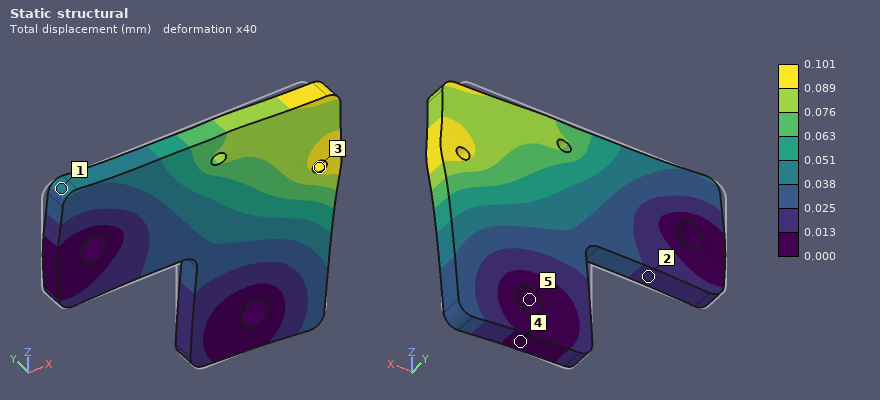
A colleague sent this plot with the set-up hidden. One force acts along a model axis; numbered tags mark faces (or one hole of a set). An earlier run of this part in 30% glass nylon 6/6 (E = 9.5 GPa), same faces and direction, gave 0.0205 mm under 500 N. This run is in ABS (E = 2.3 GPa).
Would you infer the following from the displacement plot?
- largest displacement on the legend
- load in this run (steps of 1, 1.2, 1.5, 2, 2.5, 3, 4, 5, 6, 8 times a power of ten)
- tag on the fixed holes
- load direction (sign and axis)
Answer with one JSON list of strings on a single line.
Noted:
["0.101 mm", "600 N", "5", "+X"]
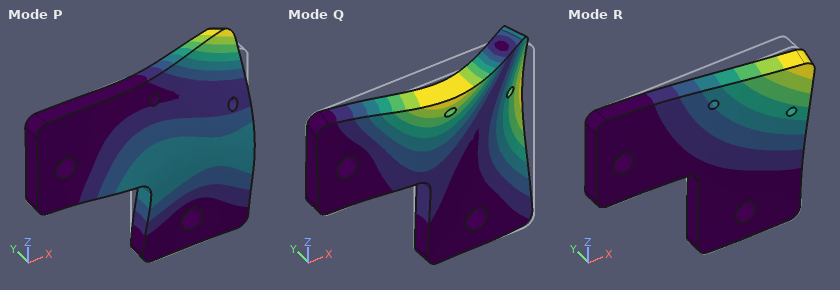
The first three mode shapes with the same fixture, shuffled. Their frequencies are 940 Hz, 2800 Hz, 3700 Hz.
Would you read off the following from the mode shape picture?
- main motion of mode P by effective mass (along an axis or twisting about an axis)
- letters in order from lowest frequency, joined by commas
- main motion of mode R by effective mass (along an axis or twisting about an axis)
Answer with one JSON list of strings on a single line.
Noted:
["along Y", "R, Q, P", "along Y"]
